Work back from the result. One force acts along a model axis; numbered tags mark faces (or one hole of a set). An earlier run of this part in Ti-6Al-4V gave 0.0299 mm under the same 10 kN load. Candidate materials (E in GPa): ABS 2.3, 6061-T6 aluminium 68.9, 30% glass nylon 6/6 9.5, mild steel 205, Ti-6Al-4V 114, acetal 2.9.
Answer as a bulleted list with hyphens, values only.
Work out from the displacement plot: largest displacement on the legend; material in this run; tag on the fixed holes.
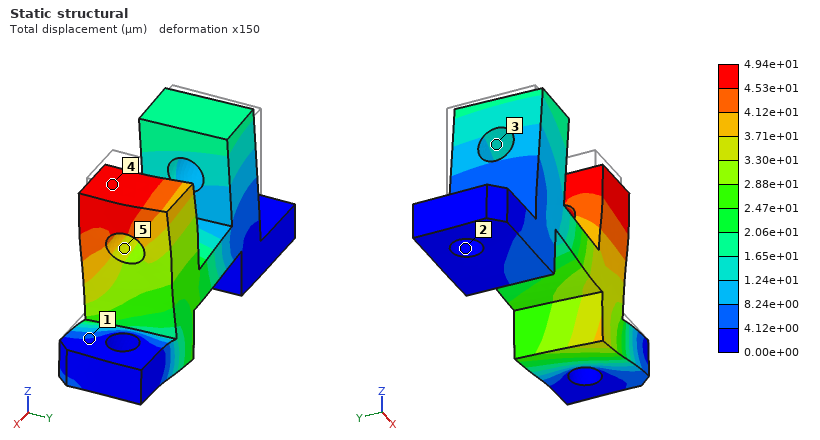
- 4.94e+01 µm
- 6061-T6 aluminium
- 2
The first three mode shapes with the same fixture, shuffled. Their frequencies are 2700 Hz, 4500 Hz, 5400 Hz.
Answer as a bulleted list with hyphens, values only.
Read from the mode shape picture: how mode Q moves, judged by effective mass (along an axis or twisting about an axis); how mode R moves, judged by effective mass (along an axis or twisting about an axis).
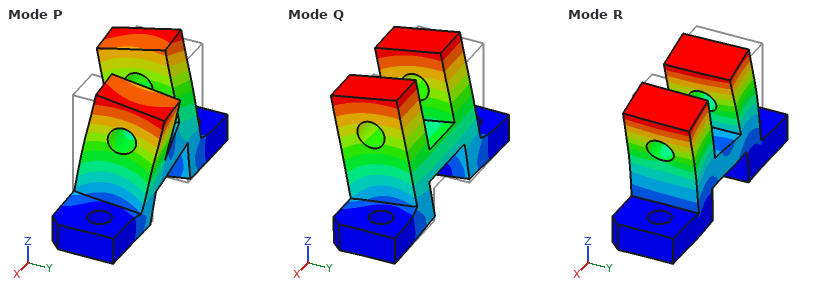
- along Y
- along X
